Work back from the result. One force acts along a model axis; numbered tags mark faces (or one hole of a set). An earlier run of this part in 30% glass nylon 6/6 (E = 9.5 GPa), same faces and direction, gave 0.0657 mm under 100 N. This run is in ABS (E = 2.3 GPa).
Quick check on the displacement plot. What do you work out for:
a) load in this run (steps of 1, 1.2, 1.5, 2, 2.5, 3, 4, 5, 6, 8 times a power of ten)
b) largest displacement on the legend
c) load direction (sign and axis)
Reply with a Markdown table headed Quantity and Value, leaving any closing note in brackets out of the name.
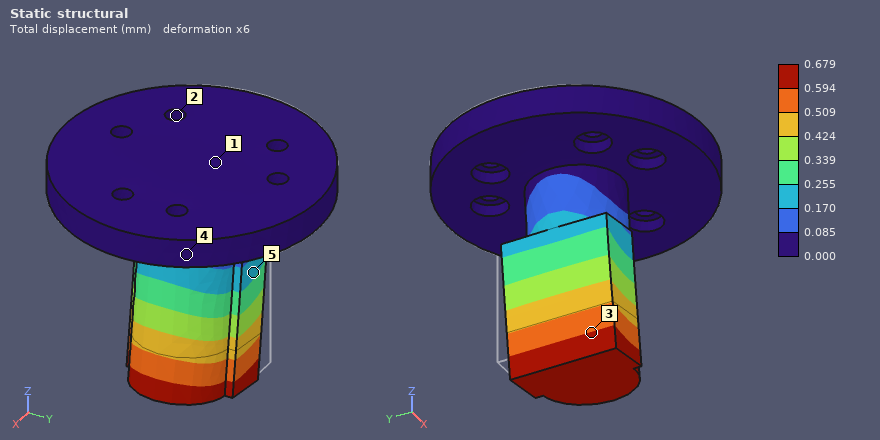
| Quantity | Value |
|---|---|
| load in this run | 250 N |
| largest displacement on the legend | 0.679 mm |
| load direction | +X |
